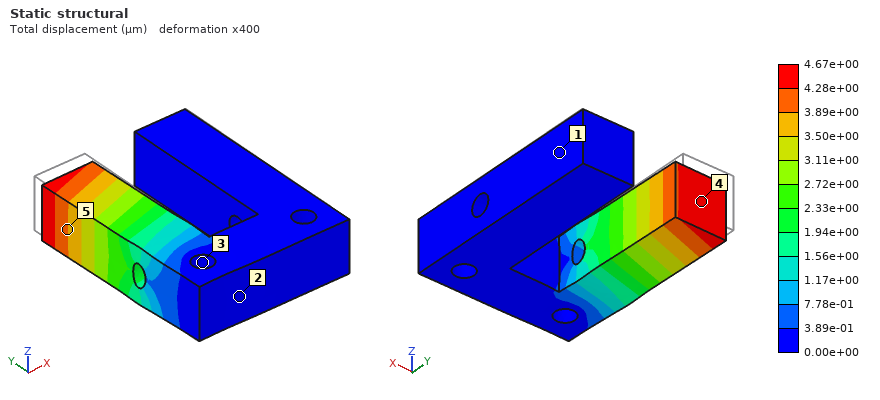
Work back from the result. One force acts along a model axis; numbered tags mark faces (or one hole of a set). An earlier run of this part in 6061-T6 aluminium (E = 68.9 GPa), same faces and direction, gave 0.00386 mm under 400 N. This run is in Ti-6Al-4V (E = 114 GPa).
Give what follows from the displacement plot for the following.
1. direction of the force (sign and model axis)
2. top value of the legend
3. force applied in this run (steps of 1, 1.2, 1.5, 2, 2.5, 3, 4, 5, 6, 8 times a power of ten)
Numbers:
-Y
4.67e+00 µm
800 N
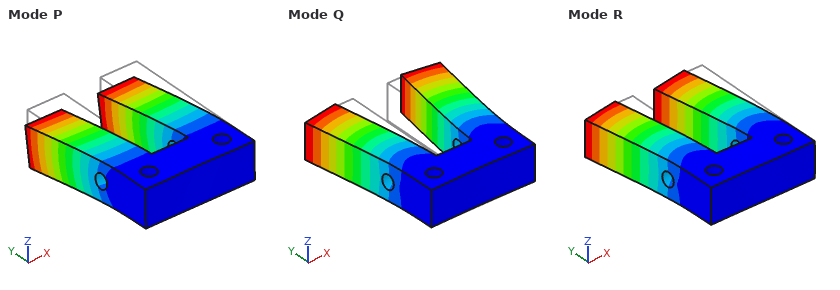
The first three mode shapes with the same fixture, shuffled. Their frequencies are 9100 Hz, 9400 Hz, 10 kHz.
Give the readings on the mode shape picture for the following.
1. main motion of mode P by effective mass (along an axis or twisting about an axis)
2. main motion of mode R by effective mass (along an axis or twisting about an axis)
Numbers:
along Z
along X
